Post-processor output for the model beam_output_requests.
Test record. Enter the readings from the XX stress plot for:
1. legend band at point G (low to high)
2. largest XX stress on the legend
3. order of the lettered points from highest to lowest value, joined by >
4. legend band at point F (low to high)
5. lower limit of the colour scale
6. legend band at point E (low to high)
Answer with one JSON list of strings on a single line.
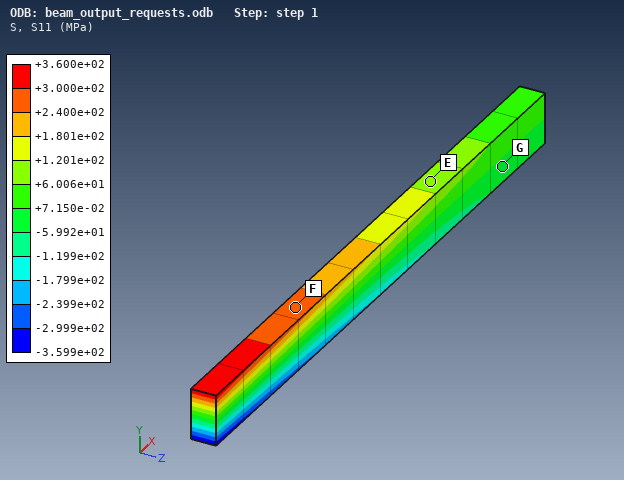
["-5.992e+01 to +7.150e-02 MPa", "+3.600e+02 MPa", "F > E > G", "+2.400e+02 to +3.000e+02 MPa", "-3.599e+02 MPa", "+6.006e+01 to +1.201e+02 MPa"]
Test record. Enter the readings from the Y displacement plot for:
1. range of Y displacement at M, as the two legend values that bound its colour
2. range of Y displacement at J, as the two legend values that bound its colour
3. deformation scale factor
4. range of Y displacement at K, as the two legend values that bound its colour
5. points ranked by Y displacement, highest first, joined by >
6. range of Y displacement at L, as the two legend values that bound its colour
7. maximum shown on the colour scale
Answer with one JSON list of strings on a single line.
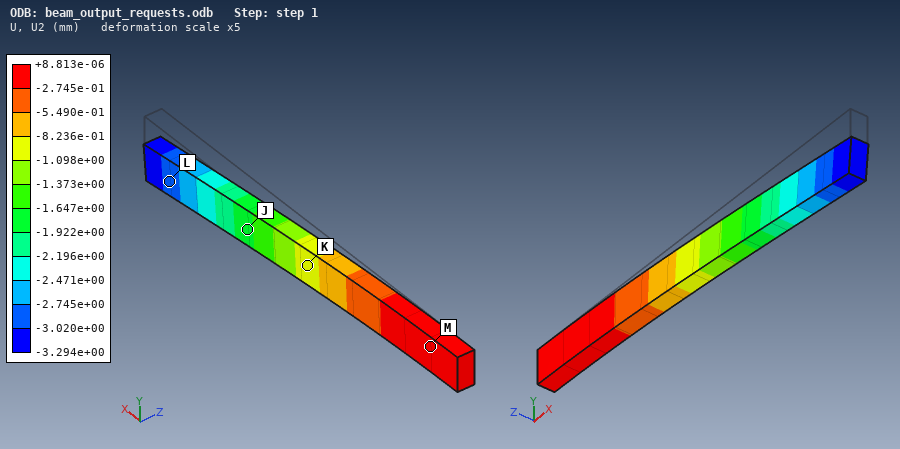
["-2.745e-01 to +8.813e-06 mm", "-1.922e+00 to -1.647e+00 mm", "5", "-1.098e+00 to -8.236e-01 mm", "M > K > J > L", "-3.020e+00 to -2.745e+00 mm", "+8.813e-06 mm"]
